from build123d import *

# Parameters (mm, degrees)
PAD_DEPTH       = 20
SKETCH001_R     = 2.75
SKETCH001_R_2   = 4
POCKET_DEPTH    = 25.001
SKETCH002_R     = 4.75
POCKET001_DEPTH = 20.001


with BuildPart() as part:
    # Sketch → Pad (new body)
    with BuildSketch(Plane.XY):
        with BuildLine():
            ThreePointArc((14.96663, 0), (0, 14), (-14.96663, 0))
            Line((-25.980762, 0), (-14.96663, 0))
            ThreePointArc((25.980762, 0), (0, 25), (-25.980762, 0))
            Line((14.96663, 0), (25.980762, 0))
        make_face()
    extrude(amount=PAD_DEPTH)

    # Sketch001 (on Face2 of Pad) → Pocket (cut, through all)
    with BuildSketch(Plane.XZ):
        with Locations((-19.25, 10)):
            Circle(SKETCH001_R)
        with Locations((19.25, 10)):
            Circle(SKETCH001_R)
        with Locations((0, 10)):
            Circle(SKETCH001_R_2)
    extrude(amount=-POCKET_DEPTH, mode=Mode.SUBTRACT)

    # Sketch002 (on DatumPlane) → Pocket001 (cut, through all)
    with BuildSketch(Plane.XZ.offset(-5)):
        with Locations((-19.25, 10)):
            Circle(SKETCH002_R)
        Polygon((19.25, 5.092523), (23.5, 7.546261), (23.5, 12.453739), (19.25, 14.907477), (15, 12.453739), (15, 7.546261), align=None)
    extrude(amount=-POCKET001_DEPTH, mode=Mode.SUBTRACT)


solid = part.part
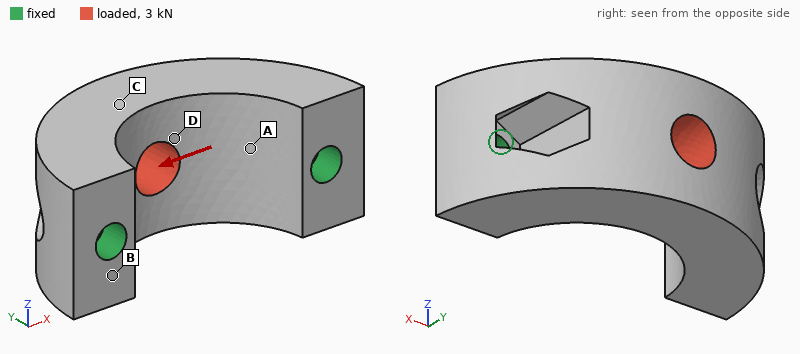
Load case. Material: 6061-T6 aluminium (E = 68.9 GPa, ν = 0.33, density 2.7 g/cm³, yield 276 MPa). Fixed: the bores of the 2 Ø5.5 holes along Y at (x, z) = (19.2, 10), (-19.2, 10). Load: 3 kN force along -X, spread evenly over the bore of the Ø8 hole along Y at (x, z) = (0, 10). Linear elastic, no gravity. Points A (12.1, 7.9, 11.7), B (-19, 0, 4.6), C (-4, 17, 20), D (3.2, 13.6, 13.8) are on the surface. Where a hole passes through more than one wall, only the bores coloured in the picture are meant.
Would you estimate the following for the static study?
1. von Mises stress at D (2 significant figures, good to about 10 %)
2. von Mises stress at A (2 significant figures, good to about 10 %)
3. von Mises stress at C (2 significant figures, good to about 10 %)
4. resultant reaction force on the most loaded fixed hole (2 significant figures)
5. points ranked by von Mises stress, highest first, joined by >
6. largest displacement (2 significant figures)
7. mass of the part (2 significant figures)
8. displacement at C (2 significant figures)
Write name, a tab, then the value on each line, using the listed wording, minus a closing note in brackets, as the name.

von Mises stress at D	31 MPa
von Mises stress at A	43 MPa
von Mises stress at C	16 MPa
resultant reaction force on the most loaded fixed hole	1.9 kN
points ranked by von Mises stress, highest first, joined by >	A > D > C > B
largest displacement	16 µm
mass of the part	31 g
displacement at C	14 µm
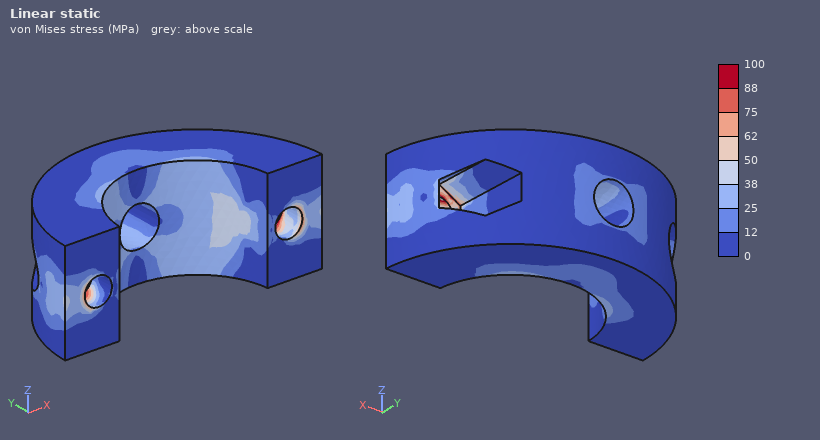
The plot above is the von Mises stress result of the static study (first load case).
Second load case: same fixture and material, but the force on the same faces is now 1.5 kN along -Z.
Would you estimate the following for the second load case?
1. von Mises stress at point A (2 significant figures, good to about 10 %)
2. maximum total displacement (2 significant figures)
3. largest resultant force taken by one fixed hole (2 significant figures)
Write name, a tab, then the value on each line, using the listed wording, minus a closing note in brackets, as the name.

von Mises stress at point A	18 MPa
maximum total displacement	51 µm
largest resultant force taken by one fixed hole	750 N
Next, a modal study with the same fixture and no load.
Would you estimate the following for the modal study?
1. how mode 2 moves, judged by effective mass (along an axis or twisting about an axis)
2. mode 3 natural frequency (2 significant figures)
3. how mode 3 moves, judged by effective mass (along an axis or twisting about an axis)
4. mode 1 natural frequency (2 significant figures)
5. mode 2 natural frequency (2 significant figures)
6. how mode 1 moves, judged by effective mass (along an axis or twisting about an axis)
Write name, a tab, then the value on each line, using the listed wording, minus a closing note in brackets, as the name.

how mode 2 moves, judged by effective mass	along X
mode 3 natural frequency	19 kHz
how mode 3 moves, judged by effective mass	twisting about Y
mode 1 natural frequency	7500 Hz
mode 2 natural frequency	16 kHz
how mode 1 moves, judged by effective mass	along Z
